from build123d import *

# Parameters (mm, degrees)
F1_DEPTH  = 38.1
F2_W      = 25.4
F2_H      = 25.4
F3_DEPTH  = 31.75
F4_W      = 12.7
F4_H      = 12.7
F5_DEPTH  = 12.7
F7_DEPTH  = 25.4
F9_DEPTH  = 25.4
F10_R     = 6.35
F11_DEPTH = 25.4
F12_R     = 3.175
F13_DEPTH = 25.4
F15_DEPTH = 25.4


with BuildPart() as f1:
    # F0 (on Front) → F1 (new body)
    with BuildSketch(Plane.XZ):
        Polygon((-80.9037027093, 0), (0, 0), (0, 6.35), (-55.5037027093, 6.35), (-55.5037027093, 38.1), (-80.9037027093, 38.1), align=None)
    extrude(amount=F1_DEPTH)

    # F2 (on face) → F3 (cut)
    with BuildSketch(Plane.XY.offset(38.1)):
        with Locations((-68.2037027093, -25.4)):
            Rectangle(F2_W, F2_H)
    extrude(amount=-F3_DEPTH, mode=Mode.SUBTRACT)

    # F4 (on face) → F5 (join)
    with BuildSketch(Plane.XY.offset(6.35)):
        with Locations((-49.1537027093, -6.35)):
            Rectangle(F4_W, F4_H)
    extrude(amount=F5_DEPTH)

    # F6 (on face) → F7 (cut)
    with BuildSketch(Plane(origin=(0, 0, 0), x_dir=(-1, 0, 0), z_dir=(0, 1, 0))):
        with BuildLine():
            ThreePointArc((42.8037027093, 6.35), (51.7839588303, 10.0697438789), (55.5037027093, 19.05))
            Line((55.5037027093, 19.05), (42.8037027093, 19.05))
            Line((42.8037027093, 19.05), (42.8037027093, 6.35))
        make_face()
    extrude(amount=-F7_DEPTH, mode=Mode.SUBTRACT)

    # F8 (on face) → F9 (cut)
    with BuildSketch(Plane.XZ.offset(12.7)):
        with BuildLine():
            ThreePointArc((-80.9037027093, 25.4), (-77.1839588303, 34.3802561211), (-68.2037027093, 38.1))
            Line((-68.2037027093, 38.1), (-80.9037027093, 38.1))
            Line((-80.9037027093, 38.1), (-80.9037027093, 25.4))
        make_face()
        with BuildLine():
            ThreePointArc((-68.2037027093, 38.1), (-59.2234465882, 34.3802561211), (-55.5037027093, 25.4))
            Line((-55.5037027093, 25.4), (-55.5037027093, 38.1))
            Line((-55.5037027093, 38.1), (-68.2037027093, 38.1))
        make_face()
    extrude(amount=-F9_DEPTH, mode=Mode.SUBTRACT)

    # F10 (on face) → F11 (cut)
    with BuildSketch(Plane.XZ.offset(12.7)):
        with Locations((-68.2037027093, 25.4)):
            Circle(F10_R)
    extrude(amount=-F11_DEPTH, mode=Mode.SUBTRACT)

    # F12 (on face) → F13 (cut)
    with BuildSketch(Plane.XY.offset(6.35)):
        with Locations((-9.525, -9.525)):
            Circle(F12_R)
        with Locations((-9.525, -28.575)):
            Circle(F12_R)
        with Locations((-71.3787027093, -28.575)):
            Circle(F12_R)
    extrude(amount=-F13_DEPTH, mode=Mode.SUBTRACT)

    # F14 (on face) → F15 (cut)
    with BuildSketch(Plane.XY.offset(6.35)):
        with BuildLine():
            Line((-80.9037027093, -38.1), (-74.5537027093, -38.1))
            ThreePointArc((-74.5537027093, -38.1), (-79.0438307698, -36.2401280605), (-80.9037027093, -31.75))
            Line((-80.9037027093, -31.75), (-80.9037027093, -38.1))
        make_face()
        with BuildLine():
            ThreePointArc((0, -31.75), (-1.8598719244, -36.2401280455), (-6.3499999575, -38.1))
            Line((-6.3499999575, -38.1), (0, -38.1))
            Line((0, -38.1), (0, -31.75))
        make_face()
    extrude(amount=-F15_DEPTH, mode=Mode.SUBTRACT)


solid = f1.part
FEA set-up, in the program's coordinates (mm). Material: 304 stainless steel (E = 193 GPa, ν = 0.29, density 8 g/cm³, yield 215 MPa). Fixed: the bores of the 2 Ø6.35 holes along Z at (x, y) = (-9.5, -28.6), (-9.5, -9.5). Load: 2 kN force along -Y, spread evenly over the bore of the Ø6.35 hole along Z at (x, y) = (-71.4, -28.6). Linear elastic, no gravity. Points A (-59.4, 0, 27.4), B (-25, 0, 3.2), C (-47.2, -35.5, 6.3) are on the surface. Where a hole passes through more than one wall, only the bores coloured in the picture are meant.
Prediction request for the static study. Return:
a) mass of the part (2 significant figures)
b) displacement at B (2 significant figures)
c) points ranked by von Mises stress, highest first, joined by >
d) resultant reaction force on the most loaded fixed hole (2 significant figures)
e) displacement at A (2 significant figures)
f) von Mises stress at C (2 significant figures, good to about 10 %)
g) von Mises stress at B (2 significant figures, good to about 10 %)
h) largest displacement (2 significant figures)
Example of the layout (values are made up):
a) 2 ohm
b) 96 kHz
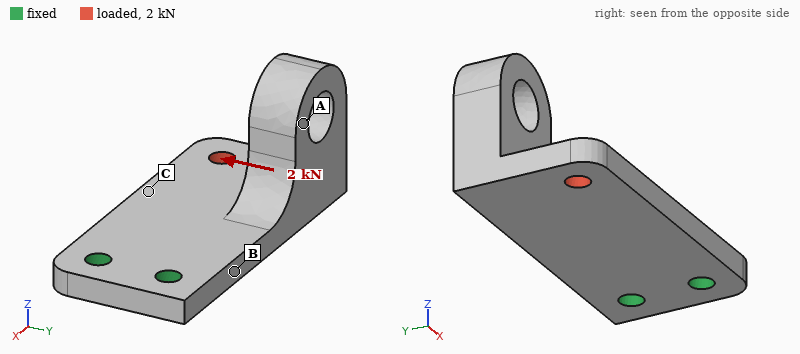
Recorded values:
a) 220 g
b) 9.3 µm
c) B > C > A
d) 5.3 kN
e) 30 µm
f) 29 MPa
g) 57 MPa
h) 49 µm
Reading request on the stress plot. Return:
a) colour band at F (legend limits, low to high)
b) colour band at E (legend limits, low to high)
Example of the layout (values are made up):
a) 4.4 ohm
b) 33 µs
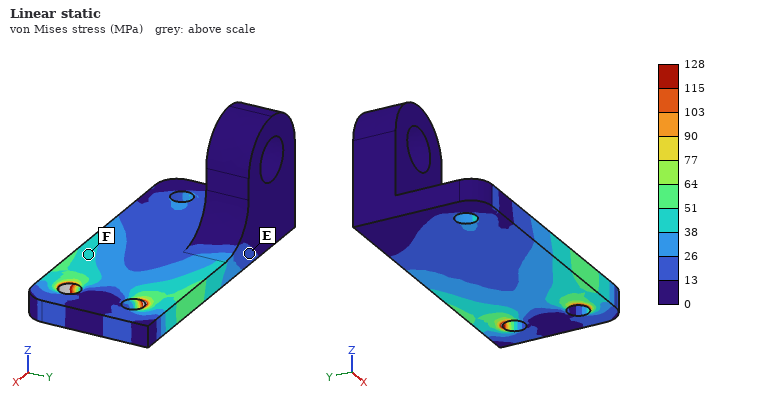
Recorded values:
a) 38 to 51 MPa
b) 13 to 26 MPa
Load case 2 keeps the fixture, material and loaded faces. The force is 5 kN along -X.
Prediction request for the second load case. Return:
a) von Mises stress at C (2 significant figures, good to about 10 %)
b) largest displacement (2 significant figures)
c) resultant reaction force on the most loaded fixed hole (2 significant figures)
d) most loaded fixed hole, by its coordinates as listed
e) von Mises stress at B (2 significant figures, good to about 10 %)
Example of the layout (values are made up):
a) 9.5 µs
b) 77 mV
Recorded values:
a) 47 MPa
b) 26 µm
c) 4.6 kN
d) (-9.5, -28.6)
e) 11 MPa
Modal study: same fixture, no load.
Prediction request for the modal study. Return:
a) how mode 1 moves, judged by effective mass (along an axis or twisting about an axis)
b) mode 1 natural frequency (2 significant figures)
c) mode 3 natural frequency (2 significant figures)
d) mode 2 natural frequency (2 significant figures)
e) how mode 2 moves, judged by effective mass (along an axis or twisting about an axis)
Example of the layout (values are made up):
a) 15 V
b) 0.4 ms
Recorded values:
a) along Z
b) 680 Hz
c) 3800 Hz
d) 1900 Hz
e) along Y
